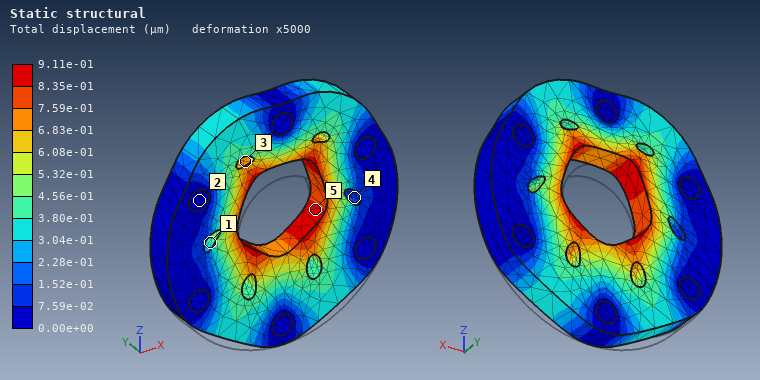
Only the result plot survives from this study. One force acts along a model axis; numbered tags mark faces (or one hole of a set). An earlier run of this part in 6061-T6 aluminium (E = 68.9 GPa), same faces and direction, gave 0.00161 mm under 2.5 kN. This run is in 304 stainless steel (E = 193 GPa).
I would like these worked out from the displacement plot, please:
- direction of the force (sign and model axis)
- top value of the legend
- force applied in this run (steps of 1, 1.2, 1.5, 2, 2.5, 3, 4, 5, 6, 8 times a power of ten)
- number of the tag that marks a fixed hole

+Z
9.11e-01 µm
4 kN
2
